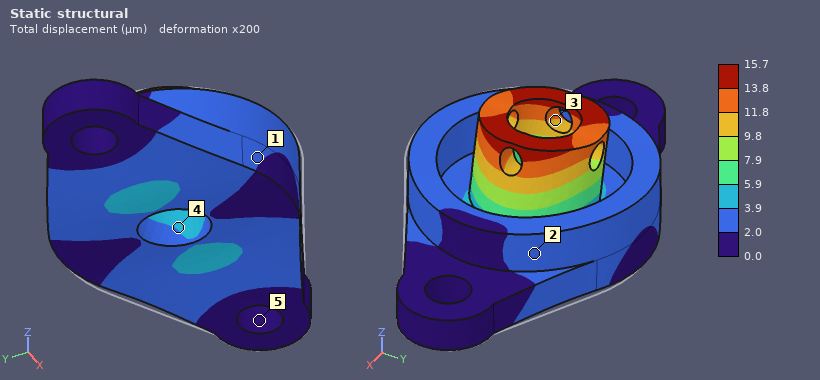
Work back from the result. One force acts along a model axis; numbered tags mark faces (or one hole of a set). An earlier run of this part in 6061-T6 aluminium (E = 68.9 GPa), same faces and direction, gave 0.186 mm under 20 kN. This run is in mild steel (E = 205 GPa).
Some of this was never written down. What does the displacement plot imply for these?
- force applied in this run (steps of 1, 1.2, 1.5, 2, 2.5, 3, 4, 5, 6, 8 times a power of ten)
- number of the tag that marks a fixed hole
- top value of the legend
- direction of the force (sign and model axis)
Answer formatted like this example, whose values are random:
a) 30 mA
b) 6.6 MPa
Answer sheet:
a) 5 kN
b) 5
c) 15.7 µm
d) -X
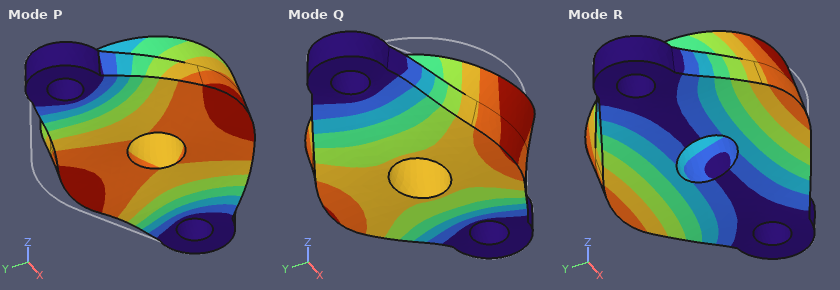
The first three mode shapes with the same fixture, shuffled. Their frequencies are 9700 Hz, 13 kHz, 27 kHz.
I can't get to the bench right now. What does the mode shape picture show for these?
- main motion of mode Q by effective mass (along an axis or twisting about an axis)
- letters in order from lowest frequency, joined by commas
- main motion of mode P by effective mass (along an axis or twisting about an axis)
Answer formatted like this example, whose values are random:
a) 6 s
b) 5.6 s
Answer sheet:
a) along Z
b) R, Q, P
c) along Y
